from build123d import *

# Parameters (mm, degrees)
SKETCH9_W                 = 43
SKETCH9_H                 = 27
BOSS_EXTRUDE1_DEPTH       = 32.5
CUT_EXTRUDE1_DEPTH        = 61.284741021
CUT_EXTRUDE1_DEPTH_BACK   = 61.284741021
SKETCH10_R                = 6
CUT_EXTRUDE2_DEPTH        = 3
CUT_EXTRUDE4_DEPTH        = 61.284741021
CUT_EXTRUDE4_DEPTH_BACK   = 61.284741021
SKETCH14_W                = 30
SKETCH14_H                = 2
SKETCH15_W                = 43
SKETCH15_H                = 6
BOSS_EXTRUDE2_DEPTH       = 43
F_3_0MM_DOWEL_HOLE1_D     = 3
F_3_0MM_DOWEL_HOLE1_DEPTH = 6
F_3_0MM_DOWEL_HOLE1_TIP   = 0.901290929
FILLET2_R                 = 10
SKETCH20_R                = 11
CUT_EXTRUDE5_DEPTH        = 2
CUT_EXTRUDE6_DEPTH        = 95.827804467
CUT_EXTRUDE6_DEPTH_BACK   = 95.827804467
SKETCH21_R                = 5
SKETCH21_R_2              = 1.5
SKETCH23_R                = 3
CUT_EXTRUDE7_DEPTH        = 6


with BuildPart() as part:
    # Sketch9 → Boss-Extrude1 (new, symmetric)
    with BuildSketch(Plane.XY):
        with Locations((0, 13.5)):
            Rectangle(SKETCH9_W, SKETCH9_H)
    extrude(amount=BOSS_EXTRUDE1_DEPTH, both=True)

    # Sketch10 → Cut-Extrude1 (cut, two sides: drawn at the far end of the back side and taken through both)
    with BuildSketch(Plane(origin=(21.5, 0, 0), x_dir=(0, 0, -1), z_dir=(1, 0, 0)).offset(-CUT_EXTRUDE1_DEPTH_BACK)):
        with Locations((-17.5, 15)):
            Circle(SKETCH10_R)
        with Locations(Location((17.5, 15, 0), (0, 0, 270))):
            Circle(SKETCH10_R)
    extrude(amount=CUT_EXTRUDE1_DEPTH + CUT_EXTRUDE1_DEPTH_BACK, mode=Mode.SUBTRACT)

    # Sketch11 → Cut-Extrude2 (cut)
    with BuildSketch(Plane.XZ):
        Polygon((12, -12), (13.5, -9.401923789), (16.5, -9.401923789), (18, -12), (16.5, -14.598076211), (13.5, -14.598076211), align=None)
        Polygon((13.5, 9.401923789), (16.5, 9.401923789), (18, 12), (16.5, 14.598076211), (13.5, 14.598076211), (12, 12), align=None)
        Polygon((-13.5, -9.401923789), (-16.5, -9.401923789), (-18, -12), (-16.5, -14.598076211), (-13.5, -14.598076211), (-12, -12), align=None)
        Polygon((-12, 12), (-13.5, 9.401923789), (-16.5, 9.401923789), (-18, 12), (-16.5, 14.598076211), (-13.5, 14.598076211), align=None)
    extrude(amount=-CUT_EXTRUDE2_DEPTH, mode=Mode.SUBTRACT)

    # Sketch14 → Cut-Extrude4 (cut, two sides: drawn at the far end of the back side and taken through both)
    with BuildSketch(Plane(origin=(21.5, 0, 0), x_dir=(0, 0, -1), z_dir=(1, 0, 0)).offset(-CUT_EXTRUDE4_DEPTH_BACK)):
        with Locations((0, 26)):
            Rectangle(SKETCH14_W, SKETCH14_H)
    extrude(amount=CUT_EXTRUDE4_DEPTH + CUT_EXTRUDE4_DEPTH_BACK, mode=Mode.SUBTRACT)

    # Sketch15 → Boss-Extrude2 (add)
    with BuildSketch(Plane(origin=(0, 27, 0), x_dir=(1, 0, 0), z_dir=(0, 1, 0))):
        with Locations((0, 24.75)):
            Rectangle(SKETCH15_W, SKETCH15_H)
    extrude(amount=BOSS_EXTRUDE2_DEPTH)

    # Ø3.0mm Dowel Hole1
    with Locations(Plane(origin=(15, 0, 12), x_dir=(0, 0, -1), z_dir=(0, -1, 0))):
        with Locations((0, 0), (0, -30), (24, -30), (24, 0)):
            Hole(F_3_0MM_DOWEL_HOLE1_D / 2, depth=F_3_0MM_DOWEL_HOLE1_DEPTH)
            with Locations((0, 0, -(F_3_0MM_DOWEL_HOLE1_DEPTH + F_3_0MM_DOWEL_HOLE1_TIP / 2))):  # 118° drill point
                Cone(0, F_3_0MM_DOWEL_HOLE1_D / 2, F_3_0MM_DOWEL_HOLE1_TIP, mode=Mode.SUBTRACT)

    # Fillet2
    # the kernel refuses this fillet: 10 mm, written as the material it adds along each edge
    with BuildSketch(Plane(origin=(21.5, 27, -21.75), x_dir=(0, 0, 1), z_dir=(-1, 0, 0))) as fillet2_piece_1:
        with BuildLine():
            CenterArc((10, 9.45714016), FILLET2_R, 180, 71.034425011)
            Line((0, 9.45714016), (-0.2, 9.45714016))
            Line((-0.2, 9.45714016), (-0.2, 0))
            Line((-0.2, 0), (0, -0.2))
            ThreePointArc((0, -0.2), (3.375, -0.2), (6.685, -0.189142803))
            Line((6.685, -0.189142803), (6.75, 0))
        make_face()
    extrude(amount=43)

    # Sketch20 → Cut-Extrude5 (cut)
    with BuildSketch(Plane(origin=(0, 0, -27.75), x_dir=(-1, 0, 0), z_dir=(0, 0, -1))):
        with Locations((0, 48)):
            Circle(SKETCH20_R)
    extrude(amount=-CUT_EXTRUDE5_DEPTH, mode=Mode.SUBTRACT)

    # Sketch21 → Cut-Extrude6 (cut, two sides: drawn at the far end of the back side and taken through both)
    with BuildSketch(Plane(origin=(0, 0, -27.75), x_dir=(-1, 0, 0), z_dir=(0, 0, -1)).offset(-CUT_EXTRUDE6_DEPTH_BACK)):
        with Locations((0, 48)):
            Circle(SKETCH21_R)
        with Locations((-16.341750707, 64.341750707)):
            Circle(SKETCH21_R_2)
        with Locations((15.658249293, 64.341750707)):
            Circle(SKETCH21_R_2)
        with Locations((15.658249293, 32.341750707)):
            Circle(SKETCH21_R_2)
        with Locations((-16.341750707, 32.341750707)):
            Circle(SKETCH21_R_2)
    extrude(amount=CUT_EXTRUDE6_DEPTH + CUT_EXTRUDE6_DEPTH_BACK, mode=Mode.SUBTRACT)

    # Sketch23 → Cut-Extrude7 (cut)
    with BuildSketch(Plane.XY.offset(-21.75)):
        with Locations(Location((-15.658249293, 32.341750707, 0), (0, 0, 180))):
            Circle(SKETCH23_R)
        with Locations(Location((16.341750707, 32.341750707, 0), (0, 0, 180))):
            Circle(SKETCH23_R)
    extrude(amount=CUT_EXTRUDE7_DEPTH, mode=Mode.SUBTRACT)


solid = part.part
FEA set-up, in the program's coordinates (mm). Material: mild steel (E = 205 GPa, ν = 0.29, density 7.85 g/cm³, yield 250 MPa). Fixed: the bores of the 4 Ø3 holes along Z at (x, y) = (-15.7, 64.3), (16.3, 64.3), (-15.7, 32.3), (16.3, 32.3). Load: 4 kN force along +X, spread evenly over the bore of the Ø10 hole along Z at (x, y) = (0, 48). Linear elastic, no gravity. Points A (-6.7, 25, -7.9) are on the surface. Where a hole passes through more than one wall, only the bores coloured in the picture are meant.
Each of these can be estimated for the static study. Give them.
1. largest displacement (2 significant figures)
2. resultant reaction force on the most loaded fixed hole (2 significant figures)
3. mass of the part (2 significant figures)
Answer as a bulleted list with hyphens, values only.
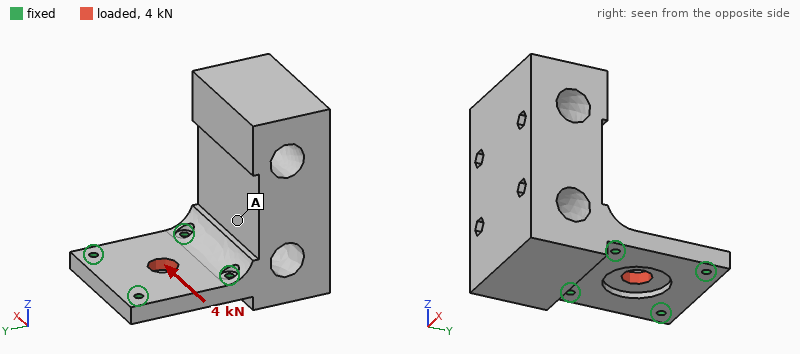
- 2.7 µm
- 1.1 kN
- 580 g
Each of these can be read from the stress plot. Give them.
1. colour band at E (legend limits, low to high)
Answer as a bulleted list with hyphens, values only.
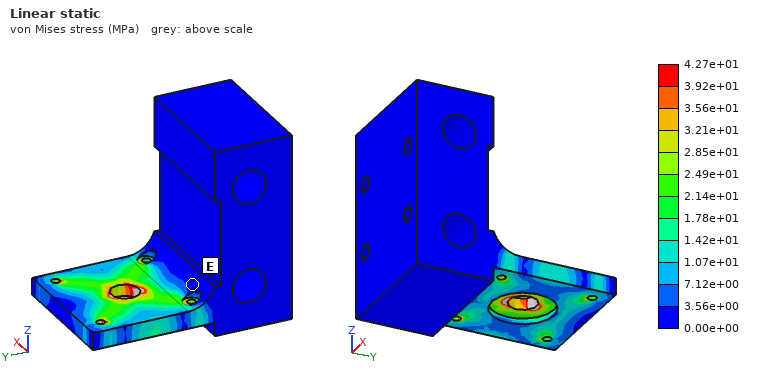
- 0.00e+00 to 3.56e+00 MPa
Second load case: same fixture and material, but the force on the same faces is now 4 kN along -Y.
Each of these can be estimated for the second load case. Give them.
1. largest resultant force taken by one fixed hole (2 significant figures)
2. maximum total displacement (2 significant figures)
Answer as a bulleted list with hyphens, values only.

- 1.2 kN
- 2.6 µm
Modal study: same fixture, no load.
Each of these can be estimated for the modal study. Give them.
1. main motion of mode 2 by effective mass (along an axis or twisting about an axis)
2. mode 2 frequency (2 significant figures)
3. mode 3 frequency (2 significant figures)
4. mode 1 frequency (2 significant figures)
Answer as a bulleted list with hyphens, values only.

- along X
- 3200 Hz
- 7300 Hz
- 960 Hz
